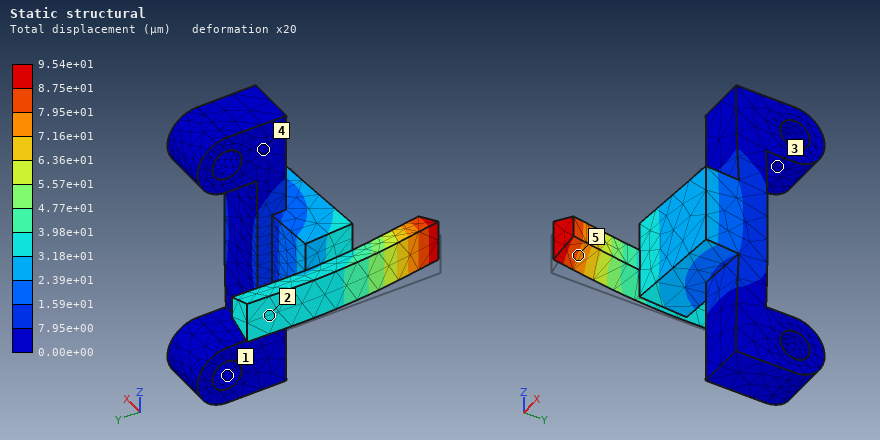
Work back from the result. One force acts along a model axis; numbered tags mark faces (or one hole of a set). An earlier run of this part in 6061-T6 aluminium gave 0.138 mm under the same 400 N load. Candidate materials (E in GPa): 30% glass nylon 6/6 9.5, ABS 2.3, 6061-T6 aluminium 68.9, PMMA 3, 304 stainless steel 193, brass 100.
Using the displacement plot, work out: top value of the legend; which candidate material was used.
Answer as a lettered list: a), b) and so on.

a) 9.54e+01 µm
b) brass
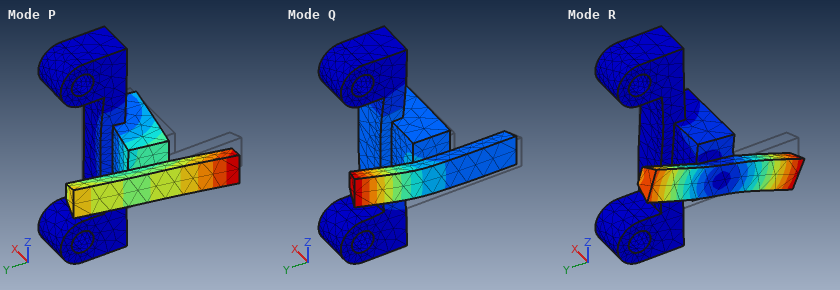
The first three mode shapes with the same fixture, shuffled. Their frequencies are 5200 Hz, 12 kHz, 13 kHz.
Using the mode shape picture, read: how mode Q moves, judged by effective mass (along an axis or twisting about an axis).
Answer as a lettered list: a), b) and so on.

a) along X
